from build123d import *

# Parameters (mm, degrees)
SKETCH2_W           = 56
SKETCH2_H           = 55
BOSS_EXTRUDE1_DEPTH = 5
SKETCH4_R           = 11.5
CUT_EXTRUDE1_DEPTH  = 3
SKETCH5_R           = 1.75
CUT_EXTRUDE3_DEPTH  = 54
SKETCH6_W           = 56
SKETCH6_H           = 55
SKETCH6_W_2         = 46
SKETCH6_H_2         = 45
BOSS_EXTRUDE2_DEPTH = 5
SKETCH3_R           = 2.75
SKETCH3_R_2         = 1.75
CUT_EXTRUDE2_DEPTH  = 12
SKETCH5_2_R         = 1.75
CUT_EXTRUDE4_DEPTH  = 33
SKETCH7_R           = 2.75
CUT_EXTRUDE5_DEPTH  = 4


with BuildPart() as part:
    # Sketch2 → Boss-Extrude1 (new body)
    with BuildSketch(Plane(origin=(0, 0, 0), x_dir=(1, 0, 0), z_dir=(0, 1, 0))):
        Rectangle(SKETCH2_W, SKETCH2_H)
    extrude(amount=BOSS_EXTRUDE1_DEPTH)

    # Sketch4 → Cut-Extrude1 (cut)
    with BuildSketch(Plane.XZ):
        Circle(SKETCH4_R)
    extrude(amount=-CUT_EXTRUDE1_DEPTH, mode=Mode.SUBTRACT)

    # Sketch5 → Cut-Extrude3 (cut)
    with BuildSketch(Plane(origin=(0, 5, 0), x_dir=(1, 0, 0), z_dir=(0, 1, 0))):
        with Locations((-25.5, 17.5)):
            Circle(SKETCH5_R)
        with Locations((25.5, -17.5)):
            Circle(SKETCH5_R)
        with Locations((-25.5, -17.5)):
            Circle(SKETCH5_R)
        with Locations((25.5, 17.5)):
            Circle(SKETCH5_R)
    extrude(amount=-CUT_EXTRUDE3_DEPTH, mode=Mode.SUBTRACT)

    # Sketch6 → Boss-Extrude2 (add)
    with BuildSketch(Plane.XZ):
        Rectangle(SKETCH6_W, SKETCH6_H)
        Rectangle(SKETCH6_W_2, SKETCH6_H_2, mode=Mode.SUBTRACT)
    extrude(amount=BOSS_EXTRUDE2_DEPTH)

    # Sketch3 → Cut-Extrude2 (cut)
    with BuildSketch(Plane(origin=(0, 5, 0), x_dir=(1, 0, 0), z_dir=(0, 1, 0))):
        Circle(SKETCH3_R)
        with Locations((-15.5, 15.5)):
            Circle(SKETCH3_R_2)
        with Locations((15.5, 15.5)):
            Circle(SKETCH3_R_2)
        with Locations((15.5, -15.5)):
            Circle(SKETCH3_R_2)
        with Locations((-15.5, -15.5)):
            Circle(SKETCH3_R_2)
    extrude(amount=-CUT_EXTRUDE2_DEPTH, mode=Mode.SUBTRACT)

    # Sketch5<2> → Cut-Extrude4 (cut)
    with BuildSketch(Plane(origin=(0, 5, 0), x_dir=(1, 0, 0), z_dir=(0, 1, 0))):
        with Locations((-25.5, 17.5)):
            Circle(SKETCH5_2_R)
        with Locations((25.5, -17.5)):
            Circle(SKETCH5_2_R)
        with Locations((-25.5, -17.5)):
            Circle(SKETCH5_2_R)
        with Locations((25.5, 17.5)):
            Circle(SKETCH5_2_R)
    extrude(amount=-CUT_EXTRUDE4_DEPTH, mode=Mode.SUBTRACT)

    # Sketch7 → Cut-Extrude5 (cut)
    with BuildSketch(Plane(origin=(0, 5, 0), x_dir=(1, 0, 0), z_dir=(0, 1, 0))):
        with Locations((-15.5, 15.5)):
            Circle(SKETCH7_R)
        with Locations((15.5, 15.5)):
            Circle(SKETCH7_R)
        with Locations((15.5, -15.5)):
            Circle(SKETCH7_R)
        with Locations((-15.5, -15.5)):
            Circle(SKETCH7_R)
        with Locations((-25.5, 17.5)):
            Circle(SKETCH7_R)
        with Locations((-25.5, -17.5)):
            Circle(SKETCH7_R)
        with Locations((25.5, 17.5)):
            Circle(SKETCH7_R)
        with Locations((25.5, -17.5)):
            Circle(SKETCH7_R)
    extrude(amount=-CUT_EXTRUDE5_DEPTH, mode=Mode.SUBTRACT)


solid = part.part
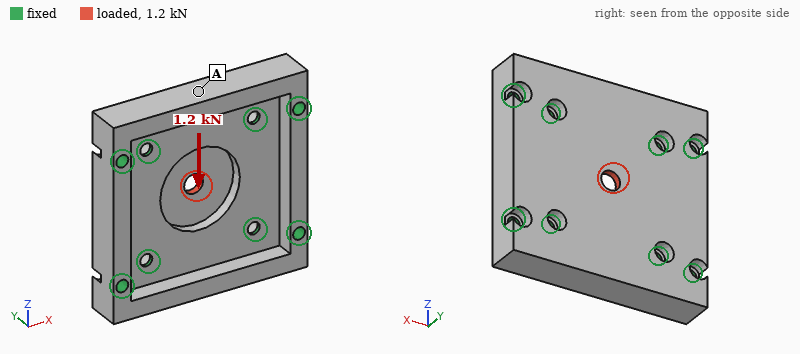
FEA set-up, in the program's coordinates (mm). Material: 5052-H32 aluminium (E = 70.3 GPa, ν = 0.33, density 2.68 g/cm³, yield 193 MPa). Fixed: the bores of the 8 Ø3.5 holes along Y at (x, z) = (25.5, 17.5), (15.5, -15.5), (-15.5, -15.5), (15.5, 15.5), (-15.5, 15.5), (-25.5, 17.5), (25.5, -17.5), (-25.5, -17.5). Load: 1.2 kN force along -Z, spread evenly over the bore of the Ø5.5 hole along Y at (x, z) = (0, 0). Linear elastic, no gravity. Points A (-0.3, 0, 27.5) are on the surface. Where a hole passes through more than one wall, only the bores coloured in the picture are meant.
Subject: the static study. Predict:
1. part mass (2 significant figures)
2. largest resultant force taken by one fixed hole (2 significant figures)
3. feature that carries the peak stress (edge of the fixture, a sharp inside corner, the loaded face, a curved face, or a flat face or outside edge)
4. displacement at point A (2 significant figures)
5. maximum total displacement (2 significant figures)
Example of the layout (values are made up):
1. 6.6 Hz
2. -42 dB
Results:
1. 49 g
2. 200 N
3. the loaded face
4. 1.8 µm
5. 5.9 µm
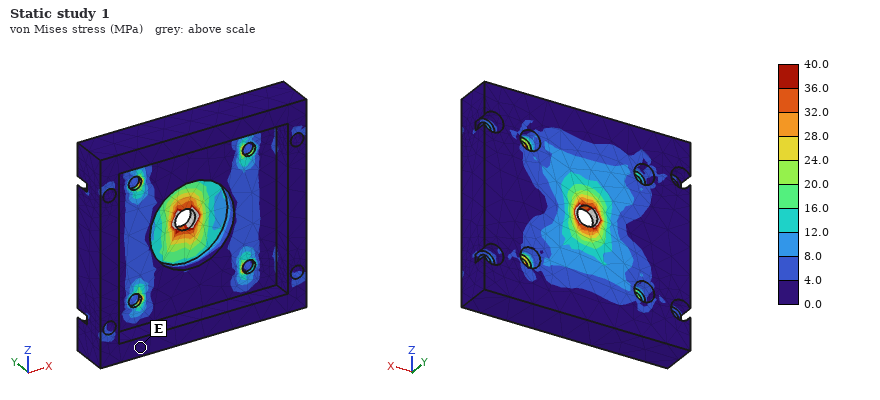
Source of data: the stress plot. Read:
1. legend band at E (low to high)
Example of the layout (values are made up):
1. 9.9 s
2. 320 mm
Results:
1. 0.0 to 4.0 MPa
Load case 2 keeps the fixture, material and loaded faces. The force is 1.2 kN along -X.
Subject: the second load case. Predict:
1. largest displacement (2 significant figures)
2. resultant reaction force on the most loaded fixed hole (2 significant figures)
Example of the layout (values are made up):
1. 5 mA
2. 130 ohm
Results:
1. 5.6 µm
2. 180 N
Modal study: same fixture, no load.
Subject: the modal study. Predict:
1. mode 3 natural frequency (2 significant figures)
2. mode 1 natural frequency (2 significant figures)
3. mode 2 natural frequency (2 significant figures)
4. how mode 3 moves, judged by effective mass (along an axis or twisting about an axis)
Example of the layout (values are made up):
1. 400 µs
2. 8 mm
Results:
1. 16 kHz
2. 14 kHz
3. 14 kHz
4. along Y
